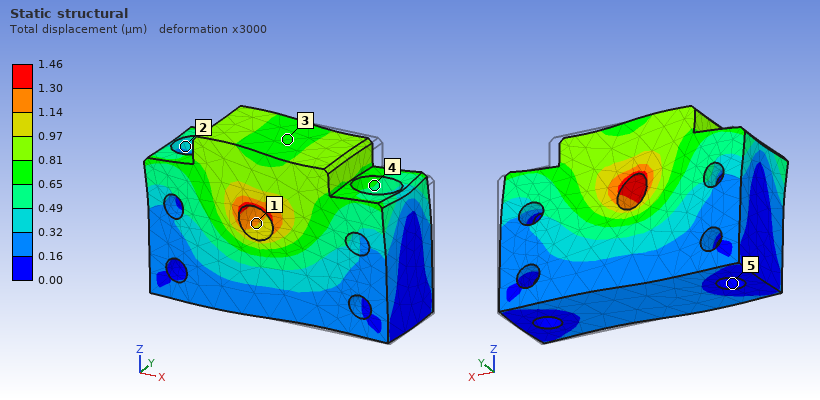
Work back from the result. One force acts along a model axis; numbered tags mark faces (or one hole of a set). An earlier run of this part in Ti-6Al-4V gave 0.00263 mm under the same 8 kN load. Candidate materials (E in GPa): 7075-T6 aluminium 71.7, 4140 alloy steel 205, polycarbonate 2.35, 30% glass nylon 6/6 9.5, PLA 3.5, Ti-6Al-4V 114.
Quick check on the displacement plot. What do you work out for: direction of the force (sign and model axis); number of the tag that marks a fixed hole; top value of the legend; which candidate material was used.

-X
5
1.46 µm
4140 alloy steel
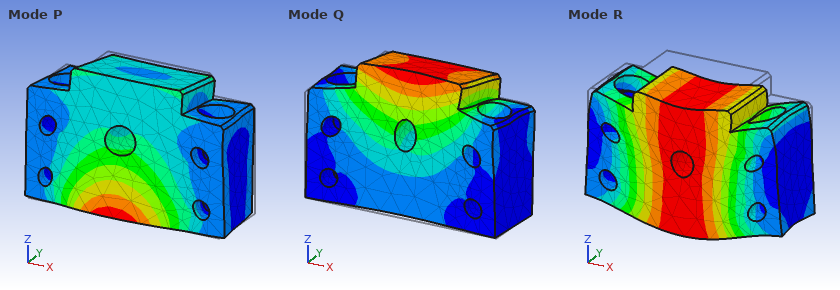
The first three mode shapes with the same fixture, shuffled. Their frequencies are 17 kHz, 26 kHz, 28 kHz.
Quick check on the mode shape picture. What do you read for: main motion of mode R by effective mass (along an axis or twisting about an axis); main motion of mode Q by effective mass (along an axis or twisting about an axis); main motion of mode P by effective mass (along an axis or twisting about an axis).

along Z
along Y
along Y
